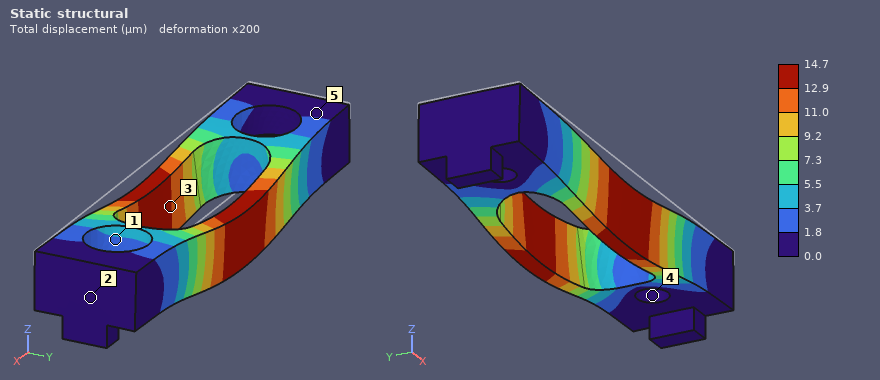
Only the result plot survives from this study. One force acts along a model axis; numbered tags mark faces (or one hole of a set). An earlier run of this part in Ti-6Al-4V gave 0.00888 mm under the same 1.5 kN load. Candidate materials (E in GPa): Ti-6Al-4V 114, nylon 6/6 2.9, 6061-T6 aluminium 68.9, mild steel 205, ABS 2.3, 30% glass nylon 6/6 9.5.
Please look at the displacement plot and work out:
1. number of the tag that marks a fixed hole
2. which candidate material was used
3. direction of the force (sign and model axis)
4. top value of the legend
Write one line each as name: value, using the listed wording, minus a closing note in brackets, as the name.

number of the tag that marks a fixed hole: 4
which candidate material was used: 6061-T6 aluminium
direction of the force: -Z
top value of the legend: 14.7 µm
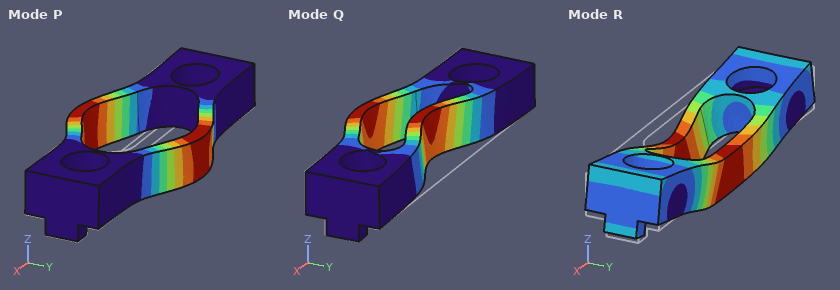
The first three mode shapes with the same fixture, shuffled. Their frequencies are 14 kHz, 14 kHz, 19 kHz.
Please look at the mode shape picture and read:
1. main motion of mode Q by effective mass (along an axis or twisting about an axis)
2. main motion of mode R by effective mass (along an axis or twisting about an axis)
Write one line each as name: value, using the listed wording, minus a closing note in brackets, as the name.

main motion of mode Q by effective mass: along Y
main motion of mode R by effective mass: along Z
